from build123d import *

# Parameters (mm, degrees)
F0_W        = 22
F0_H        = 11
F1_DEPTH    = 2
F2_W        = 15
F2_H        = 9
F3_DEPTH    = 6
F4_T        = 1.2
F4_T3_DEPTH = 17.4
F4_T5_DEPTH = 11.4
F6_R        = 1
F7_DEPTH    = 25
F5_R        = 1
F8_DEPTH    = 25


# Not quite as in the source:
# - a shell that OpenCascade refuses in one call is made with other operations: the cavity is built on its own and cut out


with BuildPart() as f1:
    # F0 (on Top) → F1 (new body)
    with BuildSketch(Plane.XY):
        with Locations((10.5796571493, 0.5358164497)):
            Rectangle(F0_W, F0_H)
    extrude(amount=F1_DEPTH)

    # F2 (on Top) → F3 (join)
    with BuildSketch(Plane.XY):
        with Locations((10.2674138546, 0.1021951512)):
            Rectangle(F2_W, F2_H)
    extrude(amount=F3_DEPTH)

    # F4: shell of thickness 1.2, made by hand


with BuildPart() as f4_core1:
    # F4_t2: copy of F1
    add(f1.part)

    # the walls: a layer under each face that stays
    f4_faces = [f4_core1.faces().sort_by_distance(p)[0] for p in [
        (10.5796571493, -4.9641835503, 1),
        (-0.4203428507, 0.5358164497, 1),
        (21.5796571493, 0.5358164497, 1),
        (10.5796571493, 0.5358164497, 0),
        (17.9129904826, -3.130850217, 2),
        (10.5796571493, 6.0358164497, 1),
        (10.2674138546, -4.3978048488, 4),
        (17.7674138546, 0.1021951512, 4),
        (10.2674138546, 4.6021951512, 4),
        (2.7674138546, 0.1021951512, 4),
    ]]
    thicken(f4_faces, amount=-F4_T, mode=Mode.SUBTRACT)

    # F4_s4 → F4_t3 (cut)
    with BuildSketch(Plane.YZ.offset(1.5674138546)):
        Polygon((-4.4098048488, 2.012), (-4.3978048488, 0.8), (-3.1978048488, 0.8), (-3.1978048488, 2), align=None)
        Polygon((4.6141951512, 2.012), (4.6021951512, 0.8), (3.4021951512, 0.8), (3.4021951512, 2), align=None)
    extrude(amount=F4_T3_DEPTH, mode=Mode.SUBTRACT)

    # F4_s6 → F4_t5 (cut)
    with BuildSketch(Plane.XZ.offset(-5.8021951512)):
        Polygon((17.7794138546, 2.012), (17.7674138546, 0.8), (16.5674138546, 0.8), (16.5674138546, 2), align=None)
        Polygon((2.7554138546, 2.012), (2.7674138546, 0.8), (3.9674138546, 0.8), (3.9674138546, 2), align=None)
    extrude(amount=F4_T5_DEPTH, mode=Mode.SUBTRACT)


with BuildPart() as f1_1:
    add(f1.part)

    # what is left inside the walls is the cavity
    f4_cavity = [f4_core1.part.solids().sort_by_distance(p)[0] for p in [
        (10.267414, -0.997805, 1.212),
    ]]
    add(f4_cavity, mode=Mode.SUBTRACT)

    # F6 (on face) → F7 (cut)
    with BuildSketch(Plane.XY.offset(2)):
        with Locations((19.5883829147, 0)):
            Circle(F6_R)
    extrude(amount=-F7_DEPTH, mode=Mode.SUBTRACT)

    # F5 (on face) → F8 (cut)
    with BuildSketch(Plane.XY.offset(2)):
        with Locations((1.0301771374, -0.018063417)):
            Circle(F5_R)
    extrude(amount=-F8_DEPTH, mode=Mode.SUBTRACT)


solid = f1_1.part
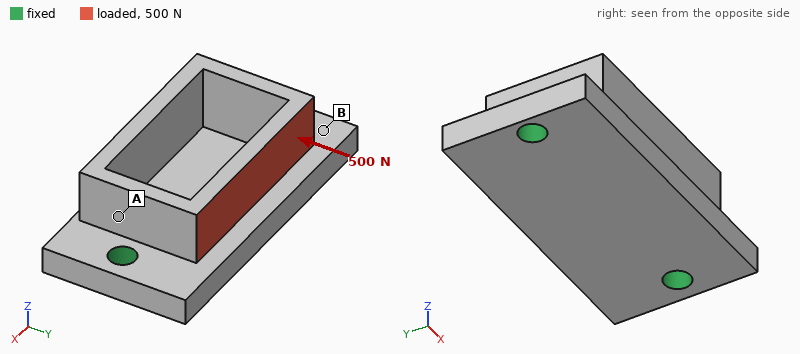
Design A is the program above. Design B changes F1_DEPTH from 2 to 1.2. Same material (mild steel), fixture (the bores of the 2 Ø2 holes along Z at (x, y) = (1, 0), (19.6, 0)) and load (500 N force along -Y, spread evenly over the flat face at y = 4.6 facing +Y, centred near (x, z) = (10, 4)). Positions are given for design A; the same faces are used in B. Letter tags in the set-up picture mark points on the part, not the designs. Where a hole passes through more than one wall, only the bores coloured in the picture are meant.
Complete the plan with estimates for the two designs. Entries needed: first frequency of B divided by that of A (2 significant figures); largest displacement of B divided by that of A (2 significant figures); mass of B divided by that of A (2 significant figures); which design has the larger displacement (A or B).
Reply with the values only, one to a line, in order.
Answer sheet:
0.63
1.5
0.87
B
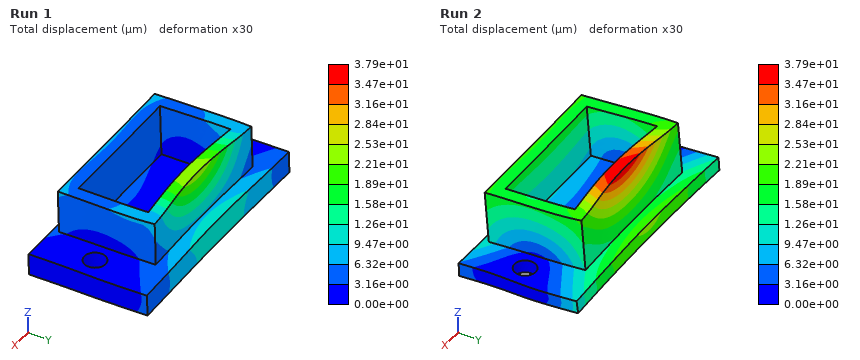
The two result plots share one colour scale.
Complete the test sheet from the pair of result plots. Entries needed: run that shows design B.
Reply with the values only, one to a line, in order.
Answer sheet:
Run 2
